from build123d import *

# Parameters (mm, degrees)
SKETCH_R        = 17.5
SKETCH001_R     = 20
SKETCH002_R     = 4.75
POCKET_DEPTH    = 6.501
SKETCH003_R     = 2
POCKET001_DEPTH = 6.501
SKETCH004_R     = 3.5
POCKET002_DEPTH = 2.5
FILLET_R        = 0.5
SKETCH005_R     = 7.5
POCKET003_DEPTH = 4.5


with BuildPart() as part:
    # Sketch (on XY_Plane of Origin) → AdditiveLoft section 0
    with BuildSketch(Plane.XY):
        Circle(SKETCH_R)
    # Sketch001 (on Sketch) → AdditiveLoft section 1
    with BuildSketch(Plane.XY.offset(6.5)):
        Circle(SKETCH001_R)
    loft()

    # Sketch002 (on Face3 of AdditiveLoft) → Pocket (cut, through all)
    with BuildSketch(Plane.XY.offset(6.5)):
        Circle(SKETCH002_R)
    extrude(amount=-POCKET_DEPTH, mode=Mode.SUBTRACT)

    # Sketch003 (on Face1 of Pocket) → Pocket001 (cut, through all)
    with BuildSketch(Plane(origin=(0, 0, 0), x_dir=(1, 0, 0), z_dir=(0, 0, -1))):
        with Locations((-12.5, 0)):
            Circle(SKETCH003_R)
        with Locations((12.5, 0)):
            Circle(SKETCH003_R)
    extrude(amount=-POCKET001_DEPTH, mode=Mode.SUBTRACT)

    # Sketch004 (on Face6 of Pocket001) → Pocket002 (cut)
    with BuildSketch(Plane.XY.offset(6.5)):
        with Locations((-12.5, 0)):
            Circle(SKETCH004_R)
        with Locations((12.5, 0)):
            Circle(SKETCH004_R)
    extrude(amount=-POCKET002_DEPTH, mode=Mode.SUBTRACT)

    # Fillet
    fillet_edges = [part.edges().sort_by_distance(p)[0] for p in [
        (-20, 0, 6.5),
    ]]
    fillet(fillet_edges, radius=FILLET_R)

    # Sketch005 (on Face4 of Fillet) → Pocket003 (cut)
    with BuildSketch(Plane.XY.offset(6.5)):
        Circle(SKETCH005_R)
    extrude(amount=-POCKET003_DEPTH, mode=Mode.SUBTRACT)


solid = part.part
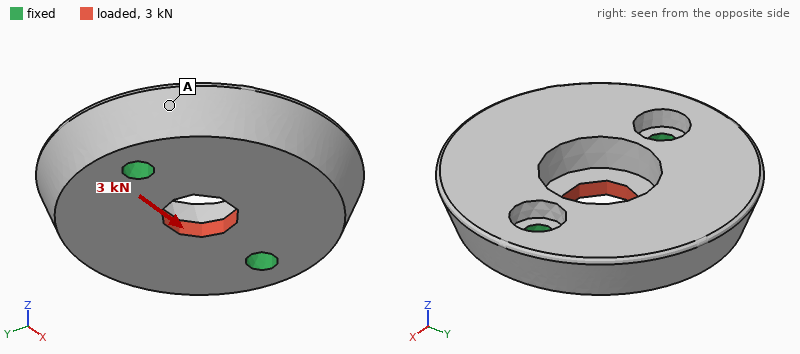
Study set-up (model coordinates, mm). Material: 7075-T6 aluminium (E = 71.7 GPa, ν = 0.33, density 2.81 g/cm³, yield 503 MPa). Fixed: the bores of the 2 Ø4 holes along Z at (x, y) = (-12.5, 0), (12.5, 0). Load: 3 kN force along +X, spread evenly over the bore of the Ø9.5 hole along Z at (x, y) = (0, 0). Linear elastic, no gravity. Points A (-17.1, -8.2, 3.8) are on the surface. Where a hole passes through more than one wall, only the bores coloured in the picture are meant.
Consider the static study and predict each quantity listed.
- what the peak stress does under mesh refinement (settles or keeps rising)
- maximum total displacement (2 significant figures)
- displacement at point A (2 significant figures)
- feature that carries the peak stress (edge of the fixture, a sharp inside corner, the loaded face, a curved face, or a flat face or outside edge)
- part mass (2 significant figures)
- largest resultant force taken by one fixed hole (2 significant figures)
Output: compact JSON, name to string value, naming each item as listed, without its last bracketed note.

{"what the peak stress does under mesh refinement": "keeps rising", "maximum total displacement": "7.0 µm", "displacement at point A": "2.1 µm", "feature that carries the peak stress": "a sharp inside corner", "part mass": "17 g", "largest resultant force taken by one fixed hole": "1.5 kN"}
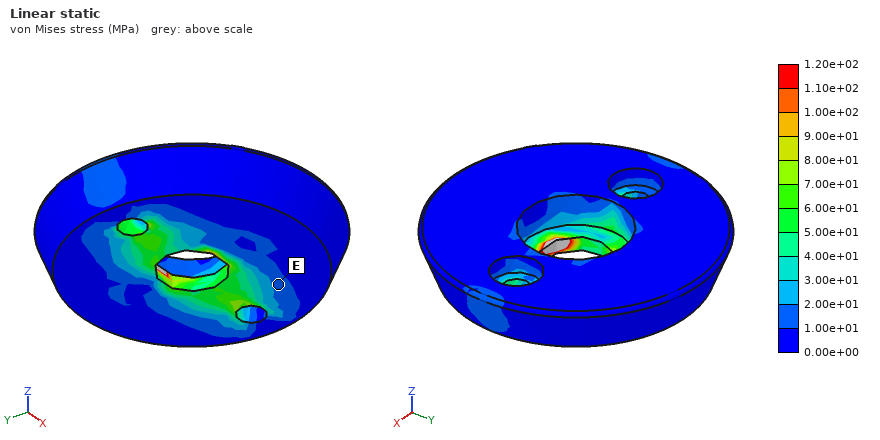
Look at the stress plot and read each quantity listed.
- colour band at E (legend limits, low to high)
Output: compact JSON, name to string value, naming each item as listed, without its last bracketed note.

{"colour band at E": "1.00e+01 to 2.00e+01 MPa"}
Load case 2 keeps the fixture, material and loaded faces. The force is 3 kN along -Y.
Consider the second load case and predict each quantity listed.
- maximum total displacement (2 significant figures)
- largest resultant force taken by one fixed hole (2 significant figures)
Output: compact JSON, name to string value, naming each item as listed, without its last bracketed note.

{"maximum total displacement": "13 µm", "largest resultant force taken by one fixed hole": "1.5 kN"}
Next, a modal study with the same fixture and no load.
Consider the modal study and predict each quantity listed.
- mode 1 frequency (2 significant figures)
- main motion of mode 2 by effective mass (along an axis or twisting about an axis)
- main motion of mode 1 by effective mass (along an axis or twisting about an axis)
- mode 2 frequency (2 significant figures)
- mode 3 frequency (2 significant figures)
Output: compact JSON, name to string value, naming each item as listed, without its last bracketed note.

{"mode 1 frequency": "9500 Hz", "main motion of mode 2 by effective mass": "along Z", "main motion of mode 1 by effective mass": "twisting about X", "mode 2 frequency": "13 kHz", "mode 3 frequency": "24 kHz"}
